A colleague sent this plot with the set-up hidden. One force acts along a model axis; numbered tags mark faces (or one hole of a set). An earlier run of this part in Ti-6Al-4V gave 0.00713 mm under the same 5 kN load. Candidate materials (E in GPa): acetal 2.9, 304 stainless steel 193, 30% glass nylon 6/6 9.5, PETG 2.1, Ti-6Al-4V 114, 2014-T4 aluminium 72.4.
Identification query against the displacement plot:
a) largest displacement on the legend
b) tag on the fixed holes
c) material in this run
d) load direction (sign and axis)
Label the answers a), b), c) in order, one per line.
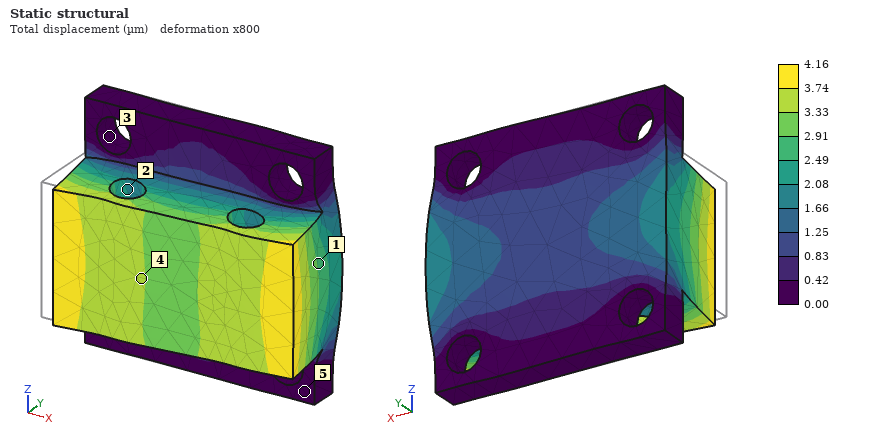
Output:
a) 4.16 µm
b) 3
c) 304 stainless steel
d) +X
